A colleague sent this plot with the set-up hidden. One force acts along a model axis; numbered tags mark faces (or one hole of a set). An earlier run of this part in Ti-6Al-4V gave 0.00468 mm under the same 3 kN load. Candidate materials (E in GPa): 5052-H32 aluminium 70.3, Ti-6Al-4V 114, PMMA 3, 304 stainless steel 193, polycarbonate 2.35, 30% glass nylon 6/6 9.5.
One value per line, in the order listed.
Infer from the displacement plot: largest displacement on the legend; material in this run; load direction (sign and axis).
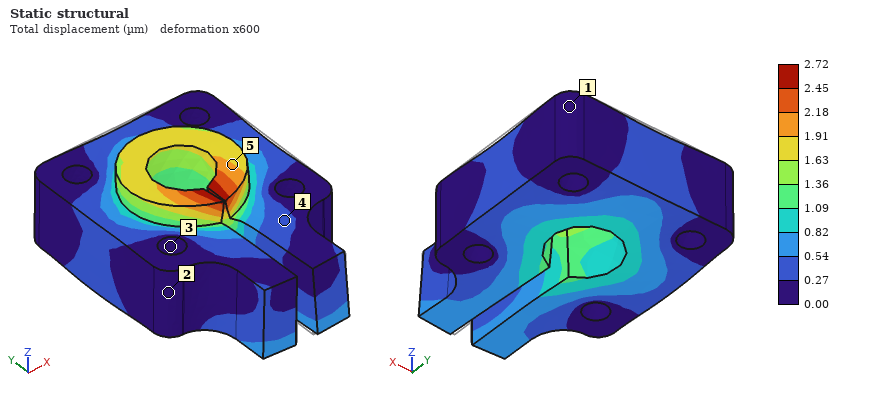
2.72 µm
304 stainless steel
-Z
